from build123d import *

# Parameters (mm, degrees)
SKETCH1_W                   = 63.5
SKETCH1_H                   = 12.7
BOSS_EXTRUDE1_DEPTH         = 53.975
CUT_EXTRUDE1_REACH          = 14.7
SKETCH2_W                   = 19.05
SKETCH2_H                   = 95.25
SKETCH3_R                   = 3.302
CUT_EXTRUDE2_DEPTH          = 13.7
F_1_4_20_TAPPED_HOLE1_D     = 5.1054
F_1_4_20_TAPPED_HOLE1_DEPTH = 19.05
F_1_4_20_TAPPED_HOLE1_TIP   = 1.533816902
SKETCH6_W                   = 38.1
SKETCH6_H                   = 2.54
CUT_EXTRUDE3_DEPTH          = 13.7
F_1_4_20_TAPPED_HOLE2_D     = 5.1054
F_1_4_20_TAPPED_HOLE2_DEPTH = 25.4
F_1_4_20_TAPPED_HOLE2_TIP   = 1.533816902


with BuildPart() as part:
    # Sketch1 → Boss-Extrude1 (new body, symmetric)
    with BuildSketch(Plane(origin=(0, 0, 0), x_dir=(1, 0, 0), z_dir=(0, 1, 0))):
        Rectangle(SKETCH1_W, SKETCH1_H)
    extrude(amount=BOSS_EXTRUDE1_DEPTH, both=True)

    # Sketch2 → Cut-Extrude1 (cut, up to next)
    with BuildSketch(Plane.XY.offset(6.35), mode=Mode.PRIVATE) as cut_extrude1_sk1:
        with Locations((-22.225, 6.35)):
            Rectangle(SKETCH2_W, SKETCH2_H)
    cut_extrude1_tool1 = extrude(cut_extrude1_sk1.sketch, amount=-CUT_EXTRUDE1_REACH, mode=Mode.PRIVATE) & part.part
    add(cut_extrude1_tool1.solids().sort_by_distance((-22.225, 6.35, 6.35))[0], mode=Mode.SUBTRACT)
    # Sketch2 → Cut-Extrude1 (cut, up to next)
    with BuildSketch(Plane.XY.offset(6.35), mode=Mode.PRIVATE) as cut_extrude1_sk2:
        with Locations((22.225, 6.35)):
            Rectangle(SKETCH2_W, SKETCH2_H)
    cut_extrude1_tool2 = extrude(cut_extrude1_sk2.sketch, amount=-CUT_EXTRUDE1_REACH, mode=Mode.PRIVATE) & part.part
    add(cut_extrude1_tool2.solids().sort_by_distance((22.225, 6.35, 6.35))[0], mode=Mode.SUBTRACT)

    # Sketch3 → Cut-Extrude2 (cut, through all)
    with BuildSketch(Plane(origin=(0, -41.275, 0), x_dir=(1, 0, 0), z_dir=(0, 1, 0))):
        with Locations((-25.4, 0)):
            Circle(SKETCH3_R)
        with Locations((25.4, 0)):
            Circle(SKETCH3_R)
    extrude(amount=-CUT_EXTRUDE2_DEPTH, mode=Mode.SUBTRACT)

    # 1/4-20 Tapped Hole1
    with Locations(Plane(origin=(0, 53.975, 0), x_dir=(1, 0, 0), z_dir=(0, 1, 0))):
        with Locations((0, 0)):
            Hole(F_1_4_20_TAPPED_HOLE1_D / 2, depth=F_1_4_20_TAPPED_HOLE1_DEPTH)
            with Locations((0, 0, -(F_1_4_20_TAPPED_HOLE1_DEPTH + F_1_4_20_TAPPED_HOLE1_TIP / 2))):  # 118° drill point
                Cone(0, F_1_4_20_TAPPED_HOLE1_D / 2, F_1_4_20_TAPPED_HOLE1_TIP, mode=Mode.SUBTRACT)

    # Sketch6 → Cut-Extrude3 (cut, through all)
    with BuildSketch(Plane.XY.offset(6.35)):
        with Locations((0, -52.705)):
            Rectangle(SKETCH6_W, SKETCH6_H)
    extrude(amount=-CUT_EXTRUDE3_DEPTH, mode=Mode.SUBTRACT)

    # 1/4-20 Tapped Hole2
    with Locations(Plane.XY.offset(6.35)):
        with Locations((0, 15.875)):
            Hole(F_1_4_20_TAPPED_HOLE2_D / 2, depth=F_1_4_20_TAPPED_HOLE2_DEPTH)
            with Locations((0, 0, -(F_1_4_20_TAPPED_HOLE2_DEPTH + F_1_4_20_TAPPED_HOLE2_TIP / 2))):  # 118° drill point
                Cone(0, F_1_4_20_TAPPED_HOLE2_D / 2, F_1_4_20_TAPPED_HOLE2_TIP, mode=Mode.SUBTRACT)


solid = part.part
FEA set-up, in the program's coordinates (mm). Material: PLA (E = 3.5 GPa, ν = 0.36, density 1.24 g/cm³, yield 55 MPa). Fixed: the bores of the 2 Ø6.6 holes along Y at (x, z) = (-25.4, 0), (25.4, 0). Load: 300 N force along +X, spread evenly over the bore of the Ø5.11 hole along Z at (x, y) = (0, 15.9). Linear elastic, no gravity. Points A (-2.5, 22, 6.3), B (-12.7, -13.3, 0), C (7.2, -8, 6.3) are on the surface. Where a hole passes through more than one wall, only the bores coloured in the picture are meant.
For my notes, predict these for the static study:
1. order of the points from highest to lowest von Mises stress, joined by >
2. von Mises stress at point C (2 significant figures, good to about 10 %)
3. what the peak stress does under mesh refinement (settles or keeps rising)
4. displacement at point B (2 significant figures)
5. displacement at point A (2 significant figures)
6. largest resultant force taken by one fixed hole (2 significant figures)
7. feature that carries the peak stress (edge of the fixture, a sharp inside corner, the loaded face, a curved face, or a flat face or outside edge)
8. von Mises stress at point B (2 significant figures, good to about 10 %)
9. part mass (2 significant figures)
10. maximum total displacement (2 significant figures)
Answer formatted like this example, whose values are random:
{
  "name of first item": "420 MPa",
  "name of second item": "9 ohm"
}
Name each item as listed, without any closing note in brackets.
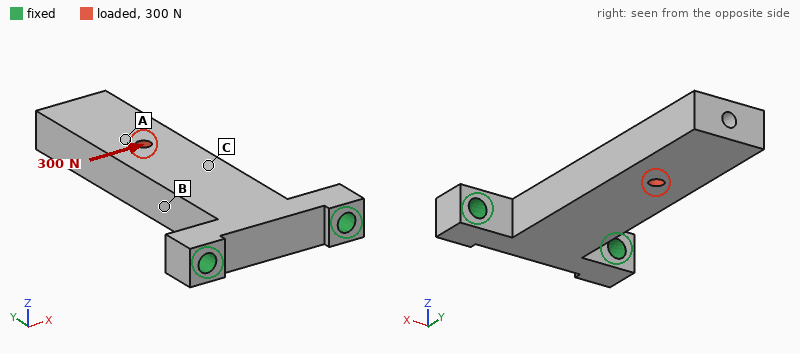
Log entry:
{
  "order of the points from highest to lowest von Mises stress, joined by >": "B > C > A",
  "von Mises stress at point C": "3.4 MPa",
  "what the peak stress does under mesh refinement": "keeps rising",
  "displacement at point B": "0.29 mm",
  "displacement at point A": "0.70 mm",
  "largest resultant force taken by one fixed hole": "550 N",
  "feature that carries the peak stress": "edge of the fixture",
  "von Mises stress at point B": "6.4 MPa",
  "part mass": "47 g",
  "maximum total displacement": "1.1 mm"
}
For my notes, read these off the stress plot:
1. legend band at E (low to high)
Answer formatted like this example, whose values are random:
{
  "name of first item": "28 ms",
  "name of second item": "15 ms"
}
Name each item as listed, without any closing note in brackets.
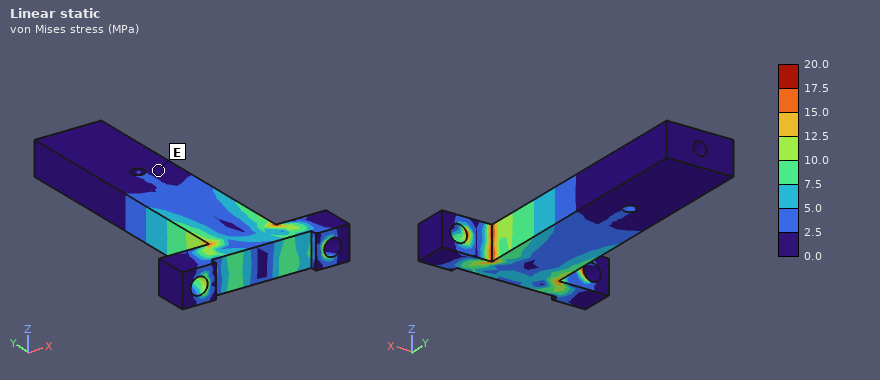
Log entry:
{
  "legend band at E": "0.0 to 2.5 MPa"
}
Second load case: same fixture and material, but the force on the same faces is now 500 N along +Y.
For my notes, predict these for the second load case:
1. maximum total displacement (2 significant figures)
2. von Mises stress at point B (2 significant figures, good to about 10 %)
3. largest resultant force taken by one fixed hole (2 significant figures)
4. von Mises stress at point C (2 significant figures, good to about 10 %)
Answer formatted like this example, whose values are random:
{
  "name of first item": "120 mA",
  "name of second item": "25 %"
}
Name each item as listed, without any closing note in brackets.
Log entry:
{
  "maximum total displacement": "65 µm",
  "von Mises stress at point B": "1.5 MPa",
  "largest resultant force taken by one fixed hole": "270 N",
  "von Mises stress at point C": "1.5 MPa"
}
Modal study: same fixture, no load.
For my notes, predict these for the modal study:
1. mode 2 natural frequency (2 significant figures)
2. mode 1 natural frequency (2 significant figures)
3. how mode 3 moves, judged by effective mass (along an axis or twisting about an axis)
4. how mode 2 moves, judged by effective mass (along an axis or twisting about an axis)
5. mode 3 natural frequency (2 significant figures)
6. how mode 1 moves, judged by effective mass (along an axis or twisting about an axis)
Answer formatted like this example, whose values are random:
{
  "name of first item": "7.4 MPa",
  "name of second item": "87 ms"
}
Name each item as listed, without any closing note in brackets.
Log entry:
{
  "mode 2 natural frequency": "570 Hz",
  "mode 1 natural frequency": "240 Hz",
  "how mode 3 moves, judged by effective mass": "along Z",
  "how mode 2 moves, judged by effective mass": "along X",
  "mode 3 natural frequency": "1600 Hz",
  "how mode 1 moves, judged by effective mass": "along Z"
}
